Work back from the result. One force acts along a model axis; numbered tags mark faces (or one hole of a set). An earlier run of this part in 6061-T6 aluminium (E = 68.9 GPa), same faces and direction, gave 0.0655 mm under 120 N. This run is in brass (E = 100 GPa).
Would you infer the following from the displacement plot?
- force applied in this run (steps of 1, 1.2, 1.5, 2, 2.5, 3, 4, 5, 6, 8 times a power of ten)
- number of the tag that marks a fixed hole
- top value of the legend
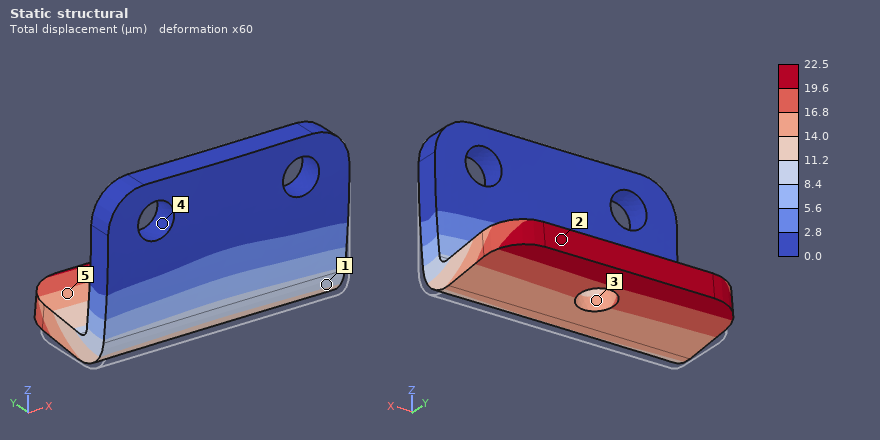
60 N
4
22.5 µm
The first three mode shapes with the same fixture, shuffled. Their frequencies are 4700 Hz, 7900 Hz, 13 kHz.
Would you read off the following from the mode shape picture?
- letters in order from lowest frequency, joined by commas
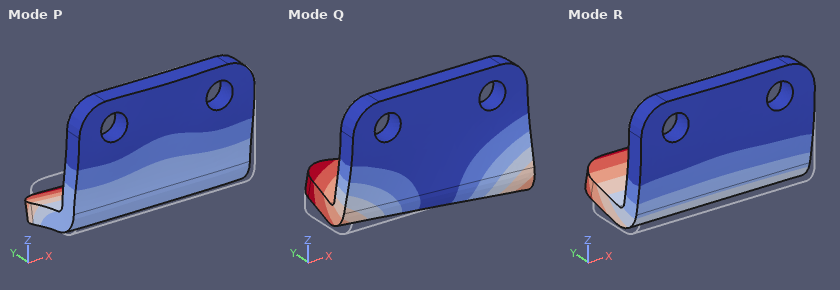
R, Q, P
